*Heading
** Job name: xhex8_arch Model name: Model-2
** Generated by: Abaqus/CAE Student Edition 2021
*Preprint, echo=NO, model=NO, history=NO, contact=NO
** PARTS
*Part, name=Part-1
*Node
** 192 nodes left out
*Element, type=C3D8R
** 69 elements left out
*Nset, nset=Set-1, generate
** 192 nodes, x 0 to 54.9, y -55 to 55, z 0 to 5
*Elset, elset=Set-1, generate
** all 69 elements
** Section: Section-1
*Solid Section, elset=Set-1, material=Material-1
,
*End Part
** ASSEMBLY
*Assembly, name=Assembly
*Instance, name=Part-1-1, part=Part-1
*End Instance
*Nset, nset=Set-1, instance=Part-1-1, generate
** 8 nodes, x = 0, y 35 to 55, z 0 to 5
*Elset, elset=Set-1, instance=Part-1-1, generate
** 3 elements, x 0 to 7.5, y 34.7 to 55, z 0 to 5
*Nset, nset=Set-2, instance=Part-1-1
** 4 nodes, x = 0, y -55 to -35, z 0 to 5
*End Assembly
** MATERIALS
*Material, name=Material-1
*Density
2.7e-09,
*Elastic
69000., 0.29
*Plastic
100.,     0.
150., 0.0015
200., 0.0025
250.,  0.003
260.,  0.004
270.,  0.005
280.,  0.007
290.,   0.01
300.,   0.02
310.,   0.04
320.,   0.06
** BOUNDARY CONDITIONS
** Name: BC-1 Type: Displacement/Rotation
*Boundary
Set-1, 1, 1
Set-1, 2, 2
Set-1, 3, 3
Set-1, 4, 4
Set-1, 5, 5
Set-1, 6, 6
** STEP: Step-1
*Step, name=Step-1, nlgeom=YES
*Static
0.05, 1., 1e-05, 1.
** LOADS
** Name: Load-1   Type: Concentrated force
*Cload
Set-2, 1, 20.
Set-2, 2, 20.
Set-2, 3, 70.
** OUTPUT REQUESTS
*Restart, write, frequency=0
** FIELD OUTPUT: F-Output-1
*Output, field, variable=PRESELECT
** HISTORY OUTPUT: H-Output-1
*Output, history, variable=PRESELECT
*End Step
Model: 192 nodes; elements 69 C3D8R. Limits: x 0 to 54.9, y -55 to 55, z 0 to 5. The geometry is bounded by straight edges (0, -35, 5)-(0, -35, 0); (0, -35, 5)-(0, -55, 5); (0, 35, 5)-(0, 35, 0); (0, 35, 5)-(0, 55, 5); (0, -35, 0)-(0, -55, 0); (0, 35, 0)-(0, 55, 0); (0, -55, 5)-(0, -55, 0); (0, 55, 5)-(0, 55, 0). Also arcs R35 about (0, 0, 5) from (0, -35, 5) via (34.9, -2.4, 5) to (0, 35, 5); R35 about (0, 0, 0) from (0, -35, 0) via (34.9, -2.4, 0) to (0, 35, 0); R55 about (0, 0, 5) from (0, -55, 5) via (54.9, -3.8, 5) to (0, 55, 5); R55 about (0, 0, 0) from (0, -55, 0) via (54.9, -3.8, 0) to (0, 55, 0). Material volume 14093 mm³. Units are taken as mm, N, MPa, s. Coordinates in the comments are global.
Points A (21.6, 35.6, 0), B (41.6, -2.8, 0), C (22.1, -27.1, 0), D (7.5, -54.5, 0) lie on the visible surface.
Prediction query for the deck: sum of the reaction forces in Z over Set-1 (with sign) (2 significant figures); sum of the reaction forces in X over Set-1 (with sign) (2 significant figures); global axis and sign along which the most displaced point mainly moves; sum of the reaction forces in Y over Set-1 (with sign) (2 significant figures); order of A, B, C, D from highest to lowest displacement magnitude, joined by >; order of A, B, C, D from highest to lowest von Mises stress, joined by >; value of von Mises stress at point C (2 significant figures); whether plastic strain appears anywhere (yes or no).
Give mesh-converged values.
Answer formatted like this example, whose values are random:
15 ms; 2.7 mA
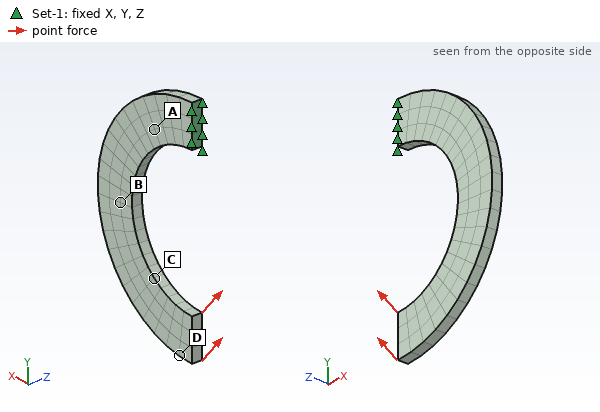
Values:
-280 N; -80 N; +Z; -80 N; D > C > B > A; A > B > C > D; 120 MPa; yes
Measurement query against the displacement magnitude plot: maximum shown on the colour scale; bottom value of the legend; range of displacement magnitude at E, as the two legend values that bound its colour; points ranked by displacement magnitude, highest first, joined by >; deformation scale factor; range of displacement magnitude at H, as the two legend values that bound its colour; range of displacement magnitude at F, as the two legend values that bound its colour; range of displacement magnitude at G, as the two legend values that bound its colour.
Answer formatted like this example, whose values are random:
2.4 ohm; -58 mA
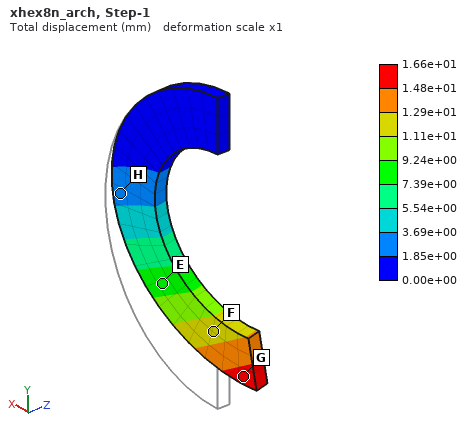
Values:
1.66e+01 mm; 0.00e+00 mm; 7.39e+00 to 9.24e+00 mm; G > F > E > H; 1; 1.85e+00 to 3.69e+00 mm; 1.11e+01 to 1.29e+01 mm; 1.48e+01 to 1.66e+01 mm
